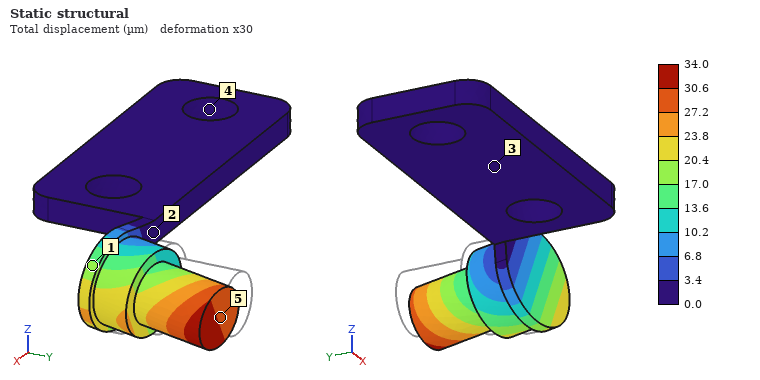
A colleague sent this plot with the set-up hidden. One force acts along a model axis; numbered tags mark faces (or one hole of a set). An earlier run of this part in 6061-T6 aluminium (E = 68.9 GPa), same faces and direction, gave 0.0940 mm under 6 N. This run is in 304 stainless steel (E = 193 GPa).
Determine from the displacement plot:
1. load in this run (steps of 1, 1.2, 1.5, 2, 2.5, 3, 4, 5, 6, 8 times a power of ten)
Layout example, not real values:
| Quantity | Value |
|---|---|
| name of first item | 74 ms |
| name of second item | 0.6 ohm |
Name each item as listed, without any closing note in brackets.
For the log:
| Quantity | Value |
|---|---|
| load in this run | 6 N |
